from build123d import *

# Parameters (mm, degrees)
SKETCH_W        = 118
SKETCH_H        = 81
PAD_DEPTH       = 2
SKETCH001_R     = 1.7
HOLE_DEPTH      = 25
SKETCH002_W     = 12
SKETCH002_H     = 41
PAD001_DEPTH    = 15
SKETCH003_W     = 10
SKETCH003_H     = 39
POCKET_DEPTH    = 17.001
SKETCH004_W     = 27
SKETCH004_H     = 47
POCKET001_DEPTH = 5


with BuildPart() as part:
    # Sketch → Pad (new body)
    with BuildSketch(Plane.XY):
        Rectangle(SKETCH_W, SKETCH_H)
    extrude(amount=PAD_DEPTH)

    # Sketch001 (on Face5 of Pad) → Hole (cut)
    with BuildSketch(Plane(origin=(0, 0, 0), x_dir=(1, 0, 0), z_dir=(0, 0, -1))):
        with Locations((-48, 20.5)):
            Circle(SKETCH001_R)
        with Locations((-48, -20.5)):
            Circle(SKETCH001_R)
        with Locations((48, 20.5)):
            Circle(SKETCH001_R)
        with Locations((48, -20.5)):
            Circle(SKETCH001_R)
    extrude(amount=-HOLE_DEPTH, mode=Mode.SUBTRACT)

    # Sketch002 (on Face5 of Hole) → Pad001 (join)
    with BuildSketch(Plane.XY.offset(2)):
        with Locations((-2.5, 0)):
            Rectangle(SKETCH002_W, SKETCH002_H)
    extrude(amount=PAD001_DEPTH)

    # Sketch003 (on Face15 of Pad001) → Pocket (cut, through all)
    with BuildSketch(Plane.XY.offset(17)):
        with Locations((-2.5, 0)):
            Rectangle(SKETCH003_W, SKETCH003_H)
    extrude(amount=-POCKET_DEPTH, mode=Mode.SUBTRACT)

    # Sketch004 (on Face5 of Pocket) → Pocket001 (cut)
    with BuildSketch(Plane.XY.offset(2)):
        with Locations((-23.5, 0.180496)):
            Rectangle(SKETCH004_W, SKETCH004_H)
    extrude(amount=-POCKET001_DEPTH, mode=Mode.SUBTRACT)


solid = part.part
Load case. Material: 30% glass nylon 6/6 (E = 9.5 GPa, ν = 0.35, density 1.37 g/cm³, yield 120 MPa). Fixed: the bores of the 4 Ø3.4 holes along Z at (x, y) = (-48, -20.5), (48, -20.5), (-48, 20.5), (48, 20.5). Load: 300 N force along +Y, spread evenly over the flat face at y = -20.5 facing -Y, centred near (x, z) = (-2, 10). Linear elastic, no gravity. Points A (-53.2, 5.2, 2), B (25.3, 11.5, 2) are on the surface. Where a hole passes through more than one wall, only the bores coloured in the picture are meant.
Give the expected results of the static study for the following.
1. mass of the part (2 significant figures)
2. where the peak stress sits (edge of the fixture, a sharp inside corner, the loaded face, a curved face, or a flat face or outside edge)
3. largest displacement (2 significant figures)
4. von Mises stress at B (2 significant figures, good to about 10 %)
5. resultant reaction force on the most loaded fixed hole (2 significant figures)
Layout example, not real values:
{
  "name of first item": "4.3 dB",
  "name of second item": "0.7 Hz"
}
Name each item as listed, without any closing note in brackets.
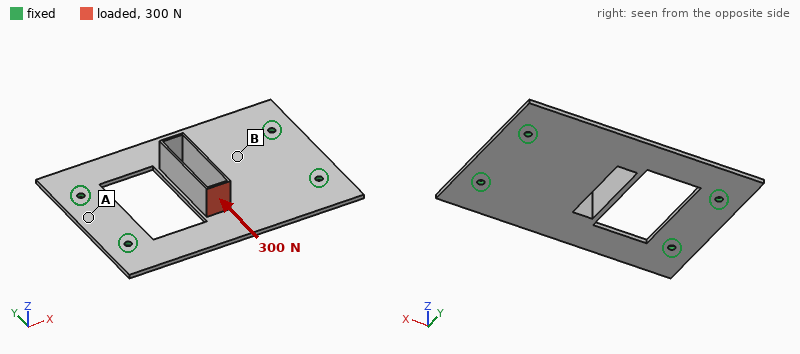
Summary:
{
  "mass of the part": "24 g",
  "where the peak stress sits": "a flat face or outside edge",
  "largest displacement": "1.4 mm",
  "von Mises stress at B": "17 MPa",
  "resultant reaction force on the most loaded fixed hole": "170 N"
}
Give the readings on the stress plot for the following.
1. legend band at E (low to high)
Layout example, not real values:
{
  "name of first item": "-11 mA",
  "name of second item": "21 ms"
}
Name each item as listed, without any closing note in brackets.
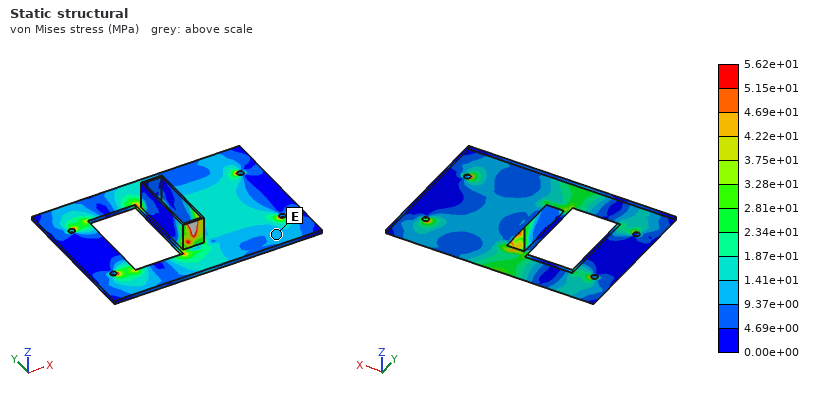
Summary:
{
  "legend band at E": "9.37e+00 to 1.41e+01 MPa"
}
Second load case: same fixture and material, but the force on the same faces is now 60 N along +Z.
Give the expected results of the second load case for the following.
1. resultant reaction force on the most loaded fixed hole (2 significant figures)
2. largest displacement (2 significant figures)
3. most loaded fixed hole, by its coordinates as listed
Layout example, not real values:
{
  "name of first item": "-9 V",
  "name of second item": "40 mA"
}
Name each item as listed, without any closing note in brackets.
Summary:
{
  "resultant reaction force on the most loaded fixed hole": "29 N",
  "largest displacement": "1.5 mm",
  "most loaded fixed hole, by its coordinates as listed": "(48, -20.5)"
}
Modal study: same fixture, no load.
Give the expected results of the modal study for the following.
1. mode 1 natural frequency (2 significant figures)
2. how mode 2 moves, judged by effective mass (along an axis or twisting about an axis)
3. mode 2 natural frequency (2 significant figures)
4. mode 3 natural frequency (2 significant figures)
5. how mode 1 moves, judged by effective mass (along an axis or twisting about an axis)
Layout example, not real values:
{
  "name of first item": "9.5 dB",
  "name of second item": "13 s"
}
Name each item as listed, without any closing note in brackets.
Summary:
{
  "mode 1 natural frequency": "460 Hz",
  "how mode 2 moves, judged by effective mass": "twisting about X",
  "mode 2 natural frequency": "580 Hz",
  "mode 3 natural frequency": "1300 Hz",
  "how mode 1 moves, judged by effective mass": "along Z"
}
